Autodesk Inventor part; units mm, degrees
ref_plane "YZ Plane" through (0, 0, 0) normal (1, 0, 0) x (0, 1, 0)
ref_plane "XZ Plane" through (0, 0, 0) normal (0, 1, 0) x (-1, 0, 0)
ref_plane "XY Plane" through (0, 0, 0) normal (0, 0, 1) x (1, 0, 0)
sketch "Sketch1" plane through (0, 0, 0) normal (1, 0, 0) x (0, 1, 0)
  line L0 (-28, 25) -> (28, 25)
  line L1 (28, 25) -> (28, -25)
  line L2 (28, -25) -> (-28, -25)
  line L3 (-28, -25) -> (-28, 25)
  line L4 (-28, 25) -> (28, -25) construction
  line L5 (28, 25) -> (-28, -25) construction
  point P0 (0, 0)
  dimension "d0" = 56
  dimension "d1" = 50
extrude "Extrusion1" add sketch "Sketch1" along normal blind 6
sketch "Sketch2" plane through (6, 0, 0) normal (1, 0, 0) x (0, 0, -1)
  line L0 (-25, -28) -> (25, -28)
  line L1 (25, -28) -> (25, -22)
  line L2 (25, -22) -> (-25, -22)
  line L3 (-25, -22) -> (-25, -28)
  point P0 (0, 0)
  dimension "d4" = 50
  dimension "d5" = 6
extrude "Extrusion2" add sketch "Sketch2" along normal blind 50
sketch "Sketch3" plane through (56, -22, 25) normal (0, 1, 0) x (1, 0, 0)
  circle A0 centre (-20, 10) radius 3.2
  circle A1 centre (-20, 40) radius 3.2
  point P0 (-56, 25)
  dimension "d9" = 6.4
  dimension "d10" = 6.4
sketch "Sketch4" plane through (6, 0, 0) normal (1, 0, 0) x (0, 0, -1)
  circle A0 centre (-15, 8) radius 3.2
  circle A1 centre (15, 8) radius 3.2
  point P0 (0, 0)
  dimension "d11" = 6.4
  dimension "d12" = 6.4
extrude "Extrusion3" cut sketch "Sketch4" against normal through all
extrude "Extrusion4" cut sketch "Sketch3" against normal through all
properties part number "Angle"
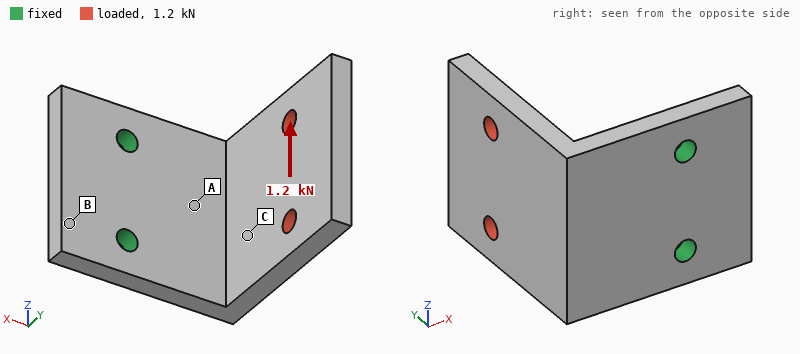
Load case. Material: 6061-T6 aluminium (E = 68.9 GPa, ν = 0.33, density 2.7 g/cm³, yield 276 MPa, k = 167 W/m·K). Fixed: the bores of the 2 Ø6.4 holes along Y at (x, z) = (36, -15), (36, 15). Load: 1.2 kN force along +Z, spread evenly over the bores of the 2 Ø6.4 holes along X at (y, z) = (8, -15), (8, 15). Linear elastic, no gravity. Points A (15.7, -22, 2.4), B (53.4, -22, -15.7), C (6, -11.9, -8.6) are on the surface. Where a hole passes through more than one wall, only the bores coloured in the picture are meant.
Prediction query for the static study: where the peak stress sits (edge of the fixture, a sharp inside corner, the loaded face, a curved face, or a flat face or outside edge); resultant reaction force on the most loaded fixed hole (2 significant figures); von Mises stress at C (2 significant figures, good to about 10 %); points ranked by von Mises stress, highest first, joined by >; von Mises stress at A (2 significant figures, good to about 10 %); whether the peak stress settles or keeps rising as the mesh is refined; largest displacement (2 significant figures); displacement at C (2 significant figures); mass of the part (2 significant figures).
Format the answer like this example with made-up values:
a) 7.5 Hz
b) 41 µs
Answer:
a) edge of the fixture
b) 1.7 kN
c) 31 MPa
d) A > C > B
e) 83 MPa
f) keeps rising
g) 0.44 mm
h) 0.12 mm
i) 84 g
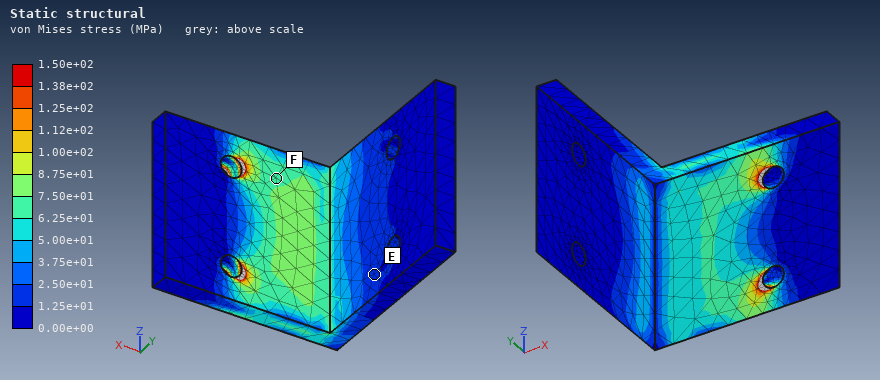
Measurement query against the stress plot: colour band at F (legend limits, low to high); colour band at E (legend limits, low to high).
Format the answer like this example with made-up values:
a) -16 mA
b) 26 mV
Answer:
a) 6.25e+01 to 7.50e+01 MPa
b) 1.25e+01 to 2.50e+01 MPa
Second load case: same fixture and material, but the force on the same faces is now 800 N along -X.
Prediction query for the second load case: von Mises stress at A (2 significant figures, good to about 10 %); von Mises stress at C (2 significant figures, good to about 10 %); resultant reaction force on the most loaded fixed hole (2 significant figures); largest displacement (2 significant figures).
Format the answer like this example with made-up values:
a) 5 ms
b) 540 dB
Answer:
a) 82 MPa
b) 49 MPa
c) 410 N
d) 0.96 mm
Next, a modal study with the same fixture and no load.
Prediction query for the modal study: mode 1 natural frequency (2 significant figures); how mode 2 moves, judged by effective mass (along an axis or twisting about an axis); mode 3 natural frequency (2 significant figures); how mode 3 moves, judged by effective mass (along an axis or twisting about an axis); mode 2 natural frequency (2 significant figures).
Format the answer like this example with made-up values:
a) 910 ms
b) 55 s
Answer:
a) 900 Hz
b) along Z
c) 2700 Hz
d) along Y
e) 1700 Hz
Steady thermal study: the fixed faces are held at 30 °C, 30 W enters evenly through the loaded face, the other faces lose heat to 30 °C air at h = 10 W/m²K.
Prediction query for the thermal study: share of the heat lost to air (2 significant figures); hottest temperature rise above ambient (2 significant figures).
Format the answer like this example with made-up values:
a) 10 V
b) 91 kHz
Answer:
a) 7.4 %
b) 39 K
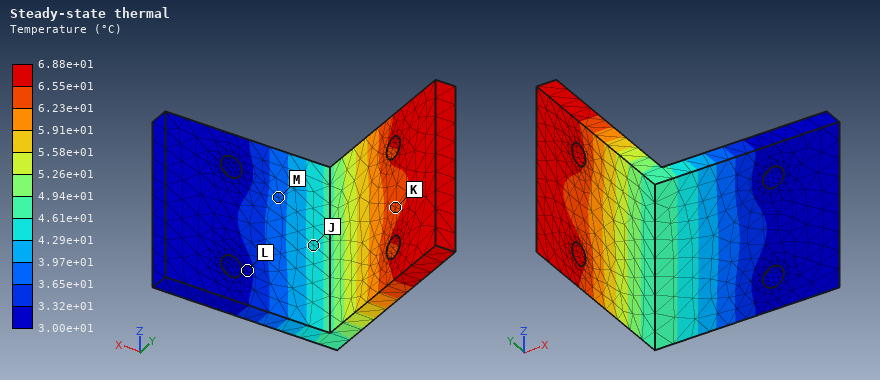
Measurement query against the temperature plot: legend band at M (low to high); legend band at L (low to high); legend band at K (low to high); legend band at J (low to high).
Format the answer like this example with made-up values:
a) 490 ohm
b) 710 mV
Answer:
a) 3.65e+01 to 3.97e+01 °C
b) 3.00e+01 to 3.32e+01 °C
c) 6.23e+01 to 6.55e+01 °C
d) 4.29e+01 to 4.61e+01 °C
